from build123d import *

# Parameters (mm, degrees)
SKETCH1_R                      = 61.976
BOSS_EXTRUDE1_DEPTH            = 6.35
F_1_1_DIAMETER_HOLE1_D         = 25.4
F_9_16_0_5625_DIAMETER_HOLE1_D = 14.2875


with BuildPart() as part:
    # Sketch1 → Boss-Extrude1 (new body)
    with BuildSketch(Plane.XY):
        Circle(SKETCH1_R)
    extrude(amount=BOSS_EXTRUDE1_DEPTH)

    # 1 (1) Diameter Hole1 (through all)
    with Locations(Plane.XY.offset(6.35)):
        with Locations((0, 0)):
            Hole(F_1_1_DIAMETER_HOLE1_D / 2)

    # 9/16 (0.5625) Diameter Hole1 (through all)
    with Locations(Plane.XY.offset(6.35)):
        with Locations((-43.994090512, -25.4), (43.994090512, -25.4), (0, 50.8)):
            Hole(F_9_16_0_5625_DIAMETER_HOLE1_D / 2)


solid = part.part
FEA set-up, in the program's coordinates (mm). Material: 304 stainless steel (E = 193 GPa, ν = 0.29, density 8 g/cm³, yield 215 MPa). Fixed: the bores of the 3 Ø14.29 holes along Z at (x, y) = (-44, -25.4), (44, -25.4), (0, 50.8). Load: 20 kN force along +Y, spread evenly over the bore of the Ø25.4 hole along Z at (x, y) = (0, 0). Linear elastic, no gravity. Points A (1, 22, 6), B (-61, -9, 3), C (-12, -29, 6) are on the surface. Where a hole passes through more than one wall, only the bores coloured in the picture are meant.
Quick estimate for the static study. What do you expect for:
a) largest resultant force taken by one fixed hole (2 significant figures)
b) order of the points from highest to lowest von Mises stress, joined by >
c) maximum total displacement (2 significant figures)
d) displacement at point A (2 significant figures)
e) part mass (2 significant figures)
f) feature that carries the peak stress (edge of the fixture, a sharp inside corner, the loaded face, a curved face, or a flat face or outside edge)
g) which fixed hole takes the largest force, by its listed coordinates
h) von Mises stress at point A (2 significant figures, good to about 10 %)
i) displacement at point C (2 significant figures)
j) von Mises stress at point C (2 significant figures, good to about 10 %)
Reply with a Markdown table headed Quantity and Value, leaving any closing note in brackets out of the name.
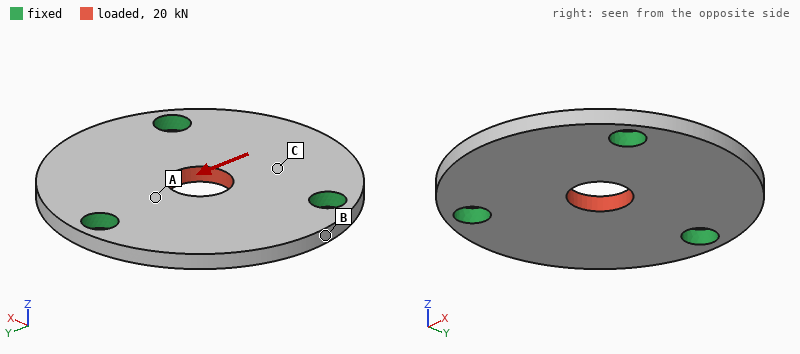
| Quantity | Value |
|---|---|
| largest resultant force taken by one fixed hole | 7.2 kN |
| order of the points from highest to lowest von Mises stress, joined by > | A > C > B |
| maximum total displacement | 11 µm |
| displacement at point A | 5.1 µm |
| part mass | 560 g |
| feature that carries the peak stress | edge of the fixture |
| which fixed hole takes the largest force, by its listed coordinates | (0, 50.8) |
| von Mises stress at point A | 45 MPa |
| displacement at point C | 7.3 µm |
| von Mises stress at point C | 23 MPa |
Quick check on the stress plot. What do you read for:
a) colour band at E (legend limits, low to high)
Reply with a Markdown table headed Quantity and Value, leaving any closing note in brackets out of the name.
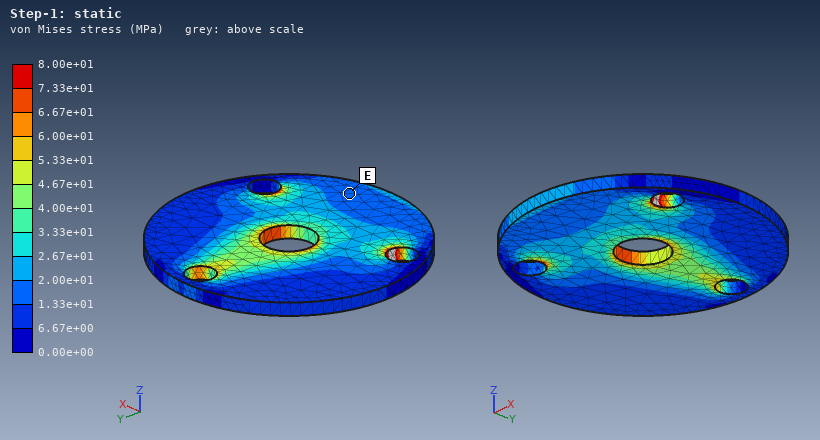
| Quantity | Value |
|---|---|
| colour band at E | 1.33e+01 to 2.00e+01 MPa |
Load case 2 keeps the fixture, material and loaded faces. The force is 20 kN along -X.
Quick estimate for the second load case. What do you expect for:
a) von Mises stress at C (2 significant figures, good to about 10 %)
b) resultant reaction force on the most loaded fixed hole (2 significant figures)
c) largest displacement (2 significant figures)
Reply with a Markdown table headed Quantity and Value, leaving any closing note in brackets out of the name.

| Quantity | Value |
|---|---|
| von Mises stress at C | 18 MPa |
| resultant reaction force on the most loaded fixed hole | 7.0 kN |
| largest displacement | 11 µm |
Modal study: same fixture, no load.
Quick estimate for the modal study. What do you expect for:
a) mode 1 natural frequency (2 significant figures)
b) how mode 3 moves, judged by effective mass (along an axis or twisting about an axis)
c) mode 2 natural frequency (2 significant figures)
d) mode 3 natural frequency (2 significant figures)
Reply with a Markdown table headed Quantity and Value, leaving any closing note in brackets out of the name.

| Quantity | Value |
|---|---|
| mode 1 natural frequency | 3300 Hz |
| how mode 3 moves, judged by effective mass | along Z |
| mode 2 natural frequency | 3300 Hz |
| mode 3 natural frequency | 3600 Hz |
